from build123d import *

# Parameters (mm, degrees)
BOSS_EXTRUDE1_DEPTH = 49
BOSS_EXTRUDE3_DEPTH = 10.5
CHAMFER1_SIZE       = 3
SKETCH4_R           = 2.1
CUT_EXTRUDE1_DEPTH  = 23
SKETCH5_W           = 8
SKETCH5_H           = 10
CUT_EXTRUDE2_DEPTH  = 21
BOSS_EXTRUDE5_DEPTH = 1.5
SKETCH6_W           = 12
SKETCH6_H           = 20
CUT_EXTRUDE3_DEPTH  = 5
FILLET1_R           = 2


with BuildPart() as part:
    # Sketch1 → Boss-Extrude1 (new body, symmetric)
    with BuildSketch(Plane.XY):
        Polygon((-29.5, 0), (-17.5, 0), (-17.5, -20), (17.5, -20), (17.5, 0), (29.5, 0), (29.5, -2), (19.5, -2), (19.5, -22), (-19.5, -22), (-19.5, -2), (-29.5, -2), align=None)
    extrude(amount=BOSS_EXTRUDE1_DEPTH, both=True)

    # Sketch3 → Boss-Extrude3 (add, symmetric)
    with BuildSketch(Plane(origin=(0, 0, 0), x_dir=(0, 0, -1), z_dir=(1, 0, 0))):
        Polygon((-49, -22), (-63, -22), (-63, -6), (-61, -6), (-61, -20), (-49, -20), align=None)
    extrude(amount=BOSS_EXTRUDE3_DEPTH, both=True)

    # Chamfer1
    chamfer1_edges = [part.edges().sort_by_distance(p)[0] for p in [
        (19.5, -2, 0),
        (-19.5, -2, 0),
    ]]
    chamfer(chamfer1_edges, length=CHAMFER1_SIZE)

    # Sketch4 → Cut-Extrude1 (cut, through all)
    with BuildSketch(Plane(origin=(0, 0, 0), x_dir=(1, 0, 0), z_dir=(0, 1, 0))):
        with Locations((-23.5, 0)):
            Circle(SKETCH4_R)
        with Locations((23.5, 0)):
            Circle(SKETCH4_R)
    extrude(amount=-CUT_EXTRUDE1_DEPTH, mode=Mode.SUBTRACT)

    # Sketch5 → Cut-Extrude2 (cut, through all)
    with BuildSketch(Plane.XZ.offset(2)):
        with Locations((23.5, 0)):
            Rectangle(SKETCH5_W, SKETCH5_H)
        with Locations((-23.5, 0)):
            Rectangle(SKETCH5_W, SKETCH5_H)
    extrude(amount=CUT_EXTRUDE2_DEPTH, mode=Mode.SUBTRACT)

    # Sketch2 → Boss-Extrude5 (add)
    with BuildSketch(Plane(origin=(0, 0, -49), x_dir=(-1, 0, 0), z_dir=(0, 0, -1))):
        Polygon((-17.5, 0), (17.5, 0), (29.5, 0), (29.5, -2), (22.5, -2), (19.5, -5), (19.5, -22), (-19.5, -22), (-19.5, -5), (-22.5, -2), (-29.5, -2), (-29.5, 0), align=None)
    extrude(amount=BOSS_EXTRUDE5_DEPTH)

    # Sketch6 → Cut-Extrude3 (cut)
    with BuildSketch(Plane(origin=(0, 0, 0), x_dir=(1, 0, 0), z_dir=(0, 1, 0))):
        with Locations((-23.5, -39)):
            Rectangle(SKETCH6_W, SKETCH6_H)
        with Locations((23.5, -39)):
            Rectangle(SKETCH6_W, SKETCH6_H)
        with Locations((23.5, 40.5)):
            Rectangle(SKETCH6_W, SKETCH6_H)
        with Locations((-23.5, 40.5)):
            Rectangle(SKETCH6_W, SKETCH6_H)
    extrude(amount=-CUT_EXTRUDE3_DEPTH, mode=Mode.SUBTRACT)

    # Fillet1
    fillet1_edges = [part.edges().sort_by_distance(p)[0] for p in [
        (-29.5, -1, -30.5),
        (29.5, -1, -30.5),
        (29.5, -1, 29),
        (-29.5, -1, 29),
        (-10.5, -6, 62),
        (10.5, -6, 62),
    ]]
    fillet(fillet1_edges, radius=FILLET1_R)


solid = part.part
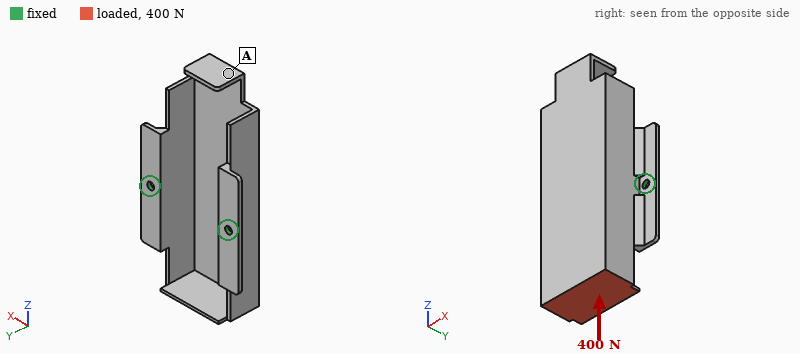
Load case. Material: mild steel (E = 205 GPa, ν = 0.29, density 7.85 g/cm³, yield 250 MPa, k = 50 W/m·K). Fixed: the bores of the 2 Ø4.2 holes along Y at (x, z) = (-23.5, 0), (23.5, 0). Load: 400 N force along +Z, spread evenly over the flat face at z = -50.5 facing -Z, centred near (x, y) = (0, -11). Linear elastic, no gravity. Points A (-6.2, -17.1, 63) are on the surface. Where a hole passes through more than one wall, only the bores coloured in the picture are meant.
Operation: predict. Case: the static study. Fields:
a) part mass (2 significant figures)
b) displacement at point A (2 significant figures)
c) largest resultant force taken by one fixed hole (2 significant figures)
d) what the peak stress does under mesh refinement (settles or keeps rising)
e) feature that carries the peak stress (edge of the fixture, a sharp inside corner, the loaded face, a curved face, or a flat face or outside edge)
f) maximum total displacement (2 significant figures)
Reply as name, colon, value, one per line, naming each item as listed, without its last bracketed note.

part mass: 160 g
displacement at point A: 77 µm
largest resultant force taken by one fixed hole: 200 N
what the peak stress does under mesh refinement: keeps rising
feature that carries the peak stress: edge of the fixture
maximum total displacement: 82 µm
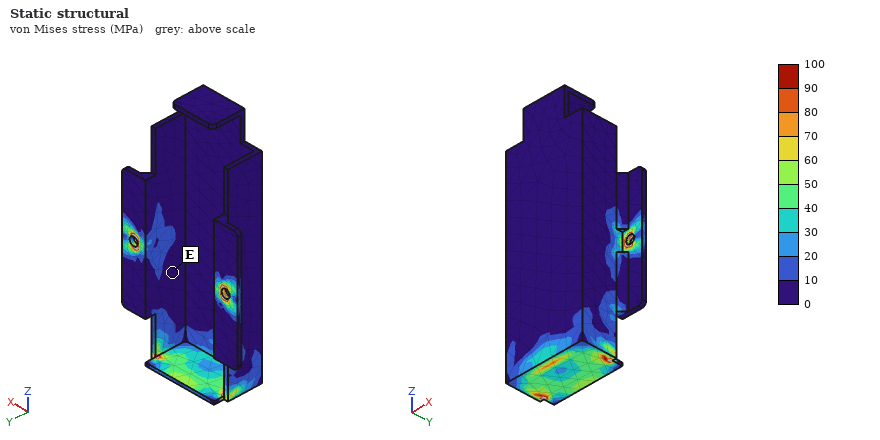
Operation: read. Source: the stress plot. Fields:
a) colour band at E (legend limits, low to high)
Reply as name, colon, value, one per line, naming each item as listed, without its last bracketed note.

colour band at E: 0 to 10 MPa
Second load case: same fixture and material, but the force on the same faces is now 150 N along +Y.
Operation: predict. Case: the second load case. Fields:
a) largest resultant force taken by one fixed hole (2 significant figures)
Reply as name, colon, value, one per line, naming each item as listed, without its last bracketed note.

largest resultant force taken by one fixed hole: 76 N
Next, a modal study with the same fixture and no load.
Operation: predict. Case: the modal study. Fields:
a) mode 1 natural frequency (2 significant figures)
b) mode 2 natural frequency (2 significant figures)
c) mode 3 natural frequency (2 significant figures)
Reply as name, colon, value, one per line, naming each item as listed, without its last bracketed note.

mode 1 natural frequency: 680 Hz
mode 2 natural frequency: 1400 Hz
mode 3 natural frequency: 1700 Hz
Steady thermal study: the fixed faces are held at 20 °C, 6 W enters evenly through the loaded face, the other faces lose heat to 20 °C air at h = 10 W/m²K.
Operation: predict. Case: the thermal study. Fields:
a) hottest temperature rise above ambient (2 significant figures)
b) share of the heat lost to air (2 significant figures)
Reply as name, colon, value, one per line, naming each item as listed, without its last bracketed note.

hottest temperature rise above ambient: 48 K
share of the heat lost to air: 41 %
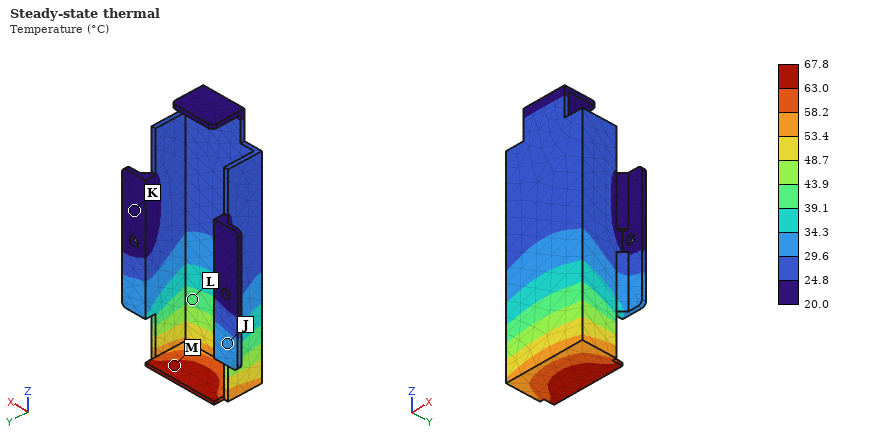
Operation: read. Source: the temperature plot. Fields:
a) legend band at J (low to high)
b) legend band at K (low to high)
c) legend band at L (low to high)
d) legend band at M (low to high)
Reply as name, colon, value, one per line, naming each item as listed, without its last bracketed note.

legend band at J: 29.6 to 34.3 °C
legend band at K: 20.0 to 24.8 °C
legend band at L: 39.1 to 43.9 °C
legend band at M: 63.0 to 67.8 °C
